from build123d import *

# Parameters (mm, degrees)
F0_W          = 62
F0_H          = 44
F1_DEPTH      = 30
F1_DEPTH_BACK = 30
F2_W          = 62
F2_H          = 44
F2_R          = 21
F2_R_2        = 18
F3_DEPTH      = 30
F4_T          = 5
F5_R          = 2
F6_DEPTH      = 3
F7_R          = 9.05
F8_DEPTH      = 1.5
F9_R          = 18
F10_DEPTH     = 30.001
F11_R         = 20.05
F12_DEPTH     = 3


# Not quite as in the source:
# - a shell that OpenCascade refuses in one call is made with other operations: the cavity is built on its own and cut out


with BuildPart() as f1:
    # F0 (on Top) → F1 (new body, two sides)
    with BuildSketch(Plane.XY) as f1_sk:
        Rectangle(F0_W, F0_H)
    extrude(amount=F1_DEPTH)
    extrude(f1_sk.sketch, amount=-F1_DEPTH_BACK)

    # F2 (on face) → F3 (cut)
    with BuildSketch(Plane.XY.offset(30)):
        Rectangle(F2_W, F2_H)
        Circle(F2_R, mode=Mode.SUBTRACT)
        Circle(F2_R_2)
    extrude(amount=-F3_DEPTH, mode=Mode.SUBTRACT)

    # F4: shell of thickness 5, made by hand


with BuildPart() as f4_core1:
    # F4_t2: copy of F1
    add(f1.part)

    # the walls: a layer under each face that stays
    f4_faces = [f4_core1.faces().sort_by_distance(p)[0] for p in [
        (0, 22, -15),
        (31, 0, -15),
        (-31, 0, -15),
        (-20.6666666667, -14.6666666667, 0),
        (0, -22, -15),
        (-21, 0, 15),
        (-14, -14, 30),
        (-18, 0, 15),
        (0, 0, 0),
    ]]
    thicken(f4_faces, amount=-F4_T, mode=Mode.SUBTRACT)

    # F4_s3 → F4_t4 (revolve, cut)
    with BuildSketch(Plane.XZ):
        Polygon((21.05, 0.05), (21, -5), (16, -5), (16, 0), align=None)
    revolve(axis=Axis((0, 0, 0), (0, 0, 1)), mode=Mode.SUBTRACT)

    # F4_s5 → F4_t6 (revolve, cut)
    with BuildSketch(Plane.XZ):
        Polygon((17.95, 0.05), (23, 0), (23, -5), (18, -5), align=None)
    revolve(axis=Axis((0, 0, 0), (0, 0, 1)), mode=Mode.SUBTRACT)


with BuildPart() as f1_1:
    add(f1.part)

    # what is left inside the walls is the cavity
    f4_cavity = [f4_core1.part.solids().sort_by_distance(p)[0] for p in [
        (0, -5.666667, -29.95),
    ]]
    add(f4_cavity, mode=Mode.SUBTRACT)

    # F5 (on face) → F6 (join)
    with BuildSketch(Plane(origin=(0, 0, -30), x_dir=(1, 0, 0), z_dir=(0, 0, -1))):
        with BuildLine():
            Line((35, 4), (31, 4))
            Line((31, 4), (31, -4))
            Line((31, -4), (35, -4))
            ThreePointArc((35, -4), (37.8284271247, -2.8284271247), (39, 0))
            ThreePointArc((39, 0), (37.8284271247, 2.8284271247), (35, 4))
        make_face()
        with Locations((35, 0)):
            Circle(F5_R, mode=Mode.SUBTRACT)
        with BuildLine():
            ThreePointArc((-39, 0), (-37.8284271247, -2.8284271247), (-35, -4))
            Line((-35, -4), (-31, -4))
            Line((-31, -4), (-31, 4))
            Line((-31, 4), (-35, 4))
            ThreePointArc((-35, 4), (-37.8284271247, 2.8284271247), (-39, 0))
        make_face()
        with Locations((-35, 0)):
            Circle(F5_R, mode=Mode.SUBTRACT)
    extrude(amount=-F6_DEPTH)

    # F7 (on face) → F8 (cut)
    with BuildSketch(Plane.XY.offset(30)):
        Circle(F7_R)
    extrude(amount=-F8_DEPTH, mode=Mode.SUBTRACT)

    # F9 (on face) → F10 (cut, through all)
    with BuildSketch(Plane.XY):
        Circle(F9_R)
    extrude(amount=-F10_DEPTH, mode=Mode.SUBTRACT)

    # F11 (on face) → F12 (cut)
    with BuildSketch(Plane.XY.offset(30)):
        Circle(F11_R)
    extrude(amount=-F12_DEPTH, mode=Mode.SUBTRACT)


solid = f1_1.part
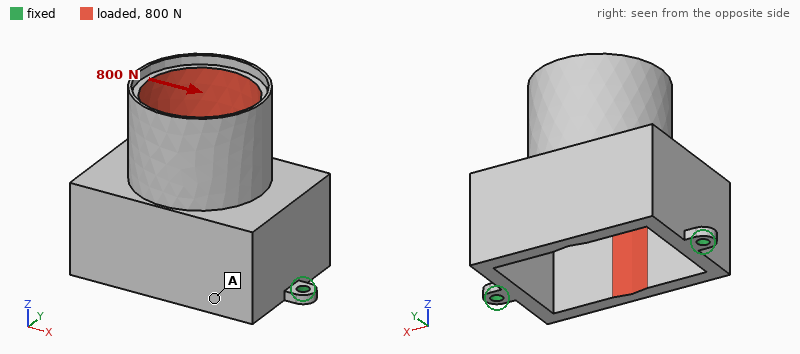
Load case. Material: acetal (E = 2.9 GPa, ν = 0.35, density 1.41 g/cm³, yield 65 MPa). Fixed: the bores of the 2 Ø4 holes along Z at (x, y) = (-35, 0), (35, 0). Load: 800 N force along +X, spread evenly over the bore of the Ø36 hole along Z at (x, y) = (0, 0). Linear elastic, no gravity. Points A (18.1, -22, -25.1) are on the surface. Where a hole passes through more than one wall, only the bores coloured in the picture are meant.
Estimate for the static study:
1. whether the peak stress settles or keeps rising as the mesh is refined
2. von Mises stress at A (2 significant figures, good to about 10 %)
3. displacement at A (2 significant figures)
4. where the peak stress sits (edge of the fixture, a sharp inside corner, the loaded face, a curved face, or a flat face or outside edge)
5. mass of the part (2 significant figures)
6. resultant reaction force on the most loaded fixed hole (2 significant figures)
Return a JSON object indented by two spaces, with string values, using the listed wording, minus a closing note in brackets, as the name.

{
  "whether the peak stress settles or keeps rising as the mesh is refined": "keeps rising",
  "von Mises stress at A": "4.2 MPa",
  "displacement at A": "0.37 mm",
  "where the peak stress sits": "edge of the fixture",
  "mass of the part": "60 g",
  "resultant reaction force on the most loaded fixed hole": "590 N"
}
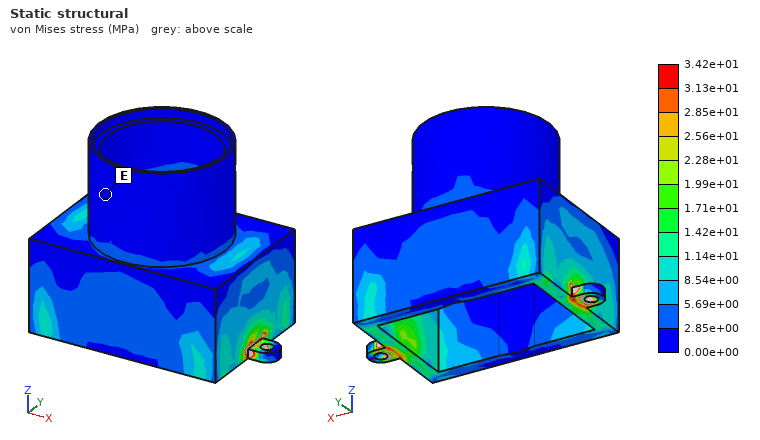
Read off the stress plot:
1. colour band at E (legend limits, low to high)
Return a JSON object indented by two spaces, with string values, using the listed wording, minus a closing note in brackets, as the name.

{
  "colour band at E": "0.00e+00 to 2.85e+00 MPa"
}
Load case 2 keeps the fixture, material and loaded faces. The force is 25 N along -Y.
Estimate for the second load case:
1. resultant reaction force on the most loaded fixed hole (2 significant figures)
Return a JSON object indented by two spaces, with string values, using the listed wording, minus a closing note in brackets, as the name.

{
  "resultant reaction force on the most loaded fixed hole": "13 N"
}
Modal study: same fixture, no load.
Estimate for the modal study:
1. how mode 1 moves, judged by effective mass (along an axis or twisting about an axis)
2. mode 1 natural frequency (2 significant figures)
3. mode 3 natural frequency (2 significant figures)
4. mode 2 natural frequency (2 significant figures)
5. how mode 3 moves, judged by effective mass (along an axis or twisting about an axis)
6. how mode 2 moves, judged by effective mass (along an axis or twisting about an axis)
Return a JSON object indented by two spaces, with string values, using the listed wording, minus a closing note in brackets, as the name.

{
  "how mode 1 moves, judged by effective mass": "along Y",
  "mode 1 natural frequency": "150 Hz",
  "mode 3 natural frequency": "980 Hz",
  "mode 2 natural frequency": "940 Hz",
  "how mode 3 moves, judged by effective mass": "twisting about Z",
  "how mode 2 moves, judged by effective mass": "along X"
}
